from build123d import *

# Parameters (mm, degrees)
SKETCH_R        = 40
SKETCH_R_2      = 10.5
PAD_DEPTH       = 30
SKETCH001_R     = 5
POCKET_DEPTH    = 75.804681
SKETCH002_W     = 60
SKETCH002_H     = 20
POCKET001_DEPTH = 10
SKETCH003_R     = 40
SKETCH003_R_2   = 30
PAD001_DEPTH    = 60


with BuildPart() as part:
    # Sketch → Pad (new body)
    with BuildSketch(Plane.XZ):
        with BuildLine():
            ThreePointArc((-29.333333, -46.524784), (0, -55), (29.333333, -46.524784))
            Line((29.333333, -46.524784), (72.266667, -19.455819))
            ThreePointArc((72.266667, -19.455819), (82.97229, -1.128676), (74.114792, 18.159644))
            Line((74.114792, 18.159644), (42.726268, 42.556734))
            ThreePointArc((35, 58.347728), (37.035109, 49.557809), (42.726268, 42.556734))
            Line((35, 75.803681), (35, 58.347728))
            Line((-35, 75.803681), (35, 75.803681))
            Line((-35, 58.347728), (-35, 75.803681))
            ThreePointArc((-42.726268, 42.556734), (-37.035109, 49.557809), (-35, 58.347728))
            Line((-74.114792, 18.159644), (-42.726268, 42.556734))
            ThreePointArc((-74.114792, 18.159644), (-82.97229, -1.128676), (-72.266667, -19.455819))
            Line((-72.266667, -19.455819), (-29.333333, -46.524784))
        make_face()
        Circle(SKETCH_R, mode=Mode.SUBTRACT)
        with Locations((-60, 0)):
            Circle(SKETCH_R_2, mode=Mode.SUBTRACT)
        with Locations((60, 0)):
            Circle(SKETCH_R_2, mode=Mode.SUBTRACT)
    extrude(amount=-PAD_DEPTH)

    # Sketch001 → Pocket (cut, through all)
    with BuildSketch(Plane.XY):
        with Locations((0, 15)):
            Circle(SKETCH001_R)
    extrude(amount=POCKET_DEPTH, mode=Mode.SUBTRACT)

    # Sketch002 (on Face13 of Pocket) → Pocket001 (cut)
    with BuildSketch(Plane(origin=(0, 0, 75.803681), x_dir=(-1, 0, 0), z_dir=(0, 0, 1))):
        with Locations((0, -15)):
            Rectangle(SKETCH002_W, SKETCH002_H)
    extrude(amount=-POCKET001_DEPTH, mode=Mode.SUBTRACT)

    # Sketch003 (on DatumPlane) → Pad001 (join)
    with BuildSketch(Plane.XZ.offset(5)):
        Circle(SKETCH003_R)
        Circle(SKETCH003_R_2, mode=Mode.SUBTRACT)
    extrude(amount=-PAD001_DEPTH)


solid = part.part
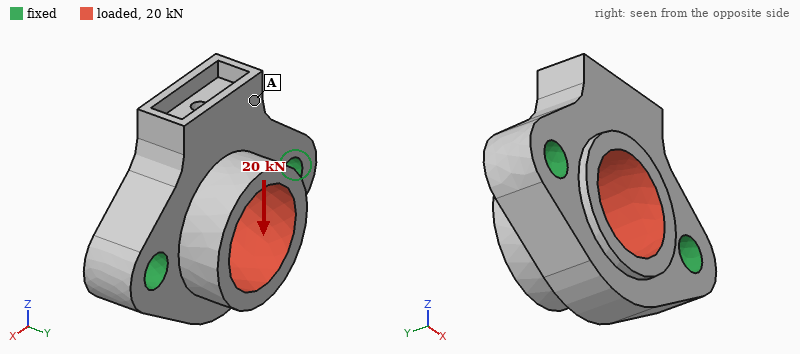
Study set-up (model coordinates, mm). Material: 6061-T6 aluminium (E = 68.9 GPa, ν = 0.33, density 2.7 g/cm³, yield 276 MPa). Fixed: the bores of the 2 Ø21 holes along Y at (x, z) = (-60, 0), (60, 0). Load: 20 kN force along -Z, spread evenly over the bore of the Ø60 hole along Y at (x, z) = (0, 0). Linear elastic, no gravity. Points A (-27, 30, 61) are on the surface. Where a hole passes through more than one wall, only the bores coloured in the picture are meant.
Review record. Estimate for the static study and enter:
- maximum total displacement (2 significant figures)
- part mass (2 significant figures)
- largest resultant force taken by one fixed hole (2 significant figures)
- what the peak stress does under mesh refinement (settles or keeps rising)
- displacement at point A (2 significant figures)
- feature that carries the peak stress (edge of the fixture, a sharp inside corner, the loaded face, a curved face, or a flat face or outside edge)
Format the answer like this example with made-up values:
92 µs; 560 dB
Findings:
24 µm; 1.0 kg; 10 kN; keeps rising; 15 µm; edge of the fixture
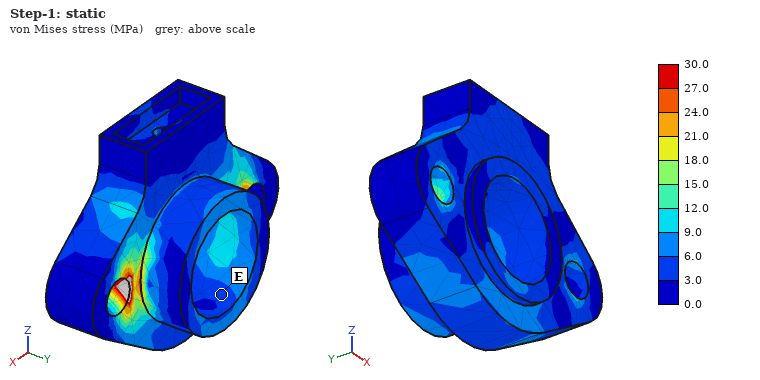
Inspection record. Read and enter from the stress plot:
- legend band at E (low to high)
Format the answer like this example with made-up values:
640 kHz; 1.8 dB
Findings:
3.0 to 6.0 MPa
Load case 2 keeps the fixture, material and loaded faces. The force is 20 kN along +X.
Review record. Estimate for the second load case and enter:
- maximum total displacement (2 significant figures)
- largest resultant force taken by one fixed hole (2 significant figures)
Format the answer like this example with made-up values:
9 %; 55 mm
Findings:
11 µm; 10 kN
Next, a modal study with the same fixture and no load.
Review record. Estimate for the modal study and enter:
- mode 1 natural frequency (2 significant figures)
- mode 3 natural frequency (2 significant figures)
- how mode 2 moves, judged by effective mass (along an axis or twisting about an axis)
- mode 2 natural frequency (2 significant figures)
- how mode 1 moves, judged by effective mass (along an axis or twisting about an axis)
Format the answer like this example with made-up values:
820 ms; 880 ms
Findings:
4100 Hz; 9100 Hz; along Y; 6100 Hz; along Y
